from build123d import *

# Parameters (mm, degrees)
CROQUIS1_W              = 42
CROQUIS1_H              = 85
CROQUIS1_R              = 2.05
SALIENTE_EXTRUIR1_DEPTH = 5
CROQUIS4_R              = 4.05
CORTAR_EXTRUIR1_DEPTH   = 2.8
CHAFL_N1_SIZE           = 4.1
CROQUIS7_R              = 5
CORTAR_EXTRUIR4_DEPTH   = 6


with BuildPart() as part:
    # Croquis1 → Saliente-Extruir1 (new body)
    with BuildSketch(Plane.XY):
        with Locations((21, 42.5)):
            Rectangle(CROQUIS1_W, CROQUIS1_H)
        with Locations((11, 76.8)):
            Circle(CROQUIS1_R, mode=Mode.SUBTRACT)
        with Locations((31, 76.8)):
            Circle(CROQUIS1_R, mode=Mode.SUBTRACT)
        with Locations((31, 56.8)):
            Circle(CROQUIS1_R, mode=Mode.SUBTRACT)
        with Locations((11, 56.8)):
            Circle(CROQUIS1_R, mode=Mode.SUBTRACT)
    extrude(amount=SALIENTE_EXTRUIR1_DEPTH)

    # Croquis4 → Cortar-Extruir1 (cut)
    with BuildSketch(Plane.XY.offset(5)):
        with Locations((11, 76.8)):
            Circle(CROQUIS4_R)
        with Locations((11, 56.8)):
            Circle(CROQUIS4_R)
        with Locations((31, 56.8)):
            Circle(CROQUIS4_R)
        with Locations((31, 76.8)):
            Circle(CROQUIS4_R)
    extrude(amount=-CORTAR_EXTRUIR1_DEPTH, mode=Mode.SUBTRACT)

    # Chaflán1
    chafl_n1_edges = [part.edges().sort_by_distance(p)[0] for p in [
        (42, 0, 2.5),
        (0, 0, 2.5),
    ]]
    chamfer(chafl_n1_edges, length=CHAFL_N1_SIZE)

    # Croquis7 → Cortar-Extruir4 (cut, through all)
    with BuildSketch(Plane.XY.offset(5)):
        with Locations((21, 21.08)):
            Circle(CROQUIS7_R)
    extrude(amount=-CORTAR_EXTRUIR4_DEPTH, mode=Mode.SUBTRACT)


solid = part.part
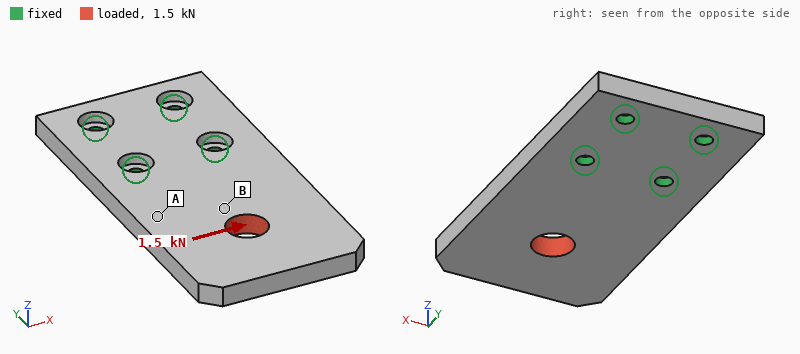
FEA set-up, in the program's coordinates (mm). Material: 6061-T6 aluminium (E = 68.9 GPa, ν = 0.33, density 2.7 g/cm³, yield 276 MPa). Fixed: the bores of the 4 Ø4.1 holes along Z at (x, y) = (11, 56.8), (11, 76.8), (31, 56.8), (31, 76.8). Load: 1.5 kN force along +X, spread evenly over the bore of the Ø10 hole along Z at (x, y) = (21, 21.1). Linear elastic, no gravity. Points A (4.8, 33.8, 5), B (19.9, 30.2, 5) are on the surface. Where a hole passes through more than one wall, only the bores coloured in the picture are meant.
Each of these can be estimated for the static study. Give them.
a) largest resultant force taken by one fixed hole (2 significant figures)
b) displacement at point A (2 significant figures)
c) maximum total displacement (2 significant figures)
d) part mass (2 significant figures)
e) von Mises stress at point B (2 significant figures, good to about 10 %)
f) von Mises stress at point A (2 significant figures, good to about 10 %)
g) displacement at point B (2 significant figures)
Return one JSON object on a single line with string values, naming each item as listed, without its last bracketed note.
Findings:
{"largest resultant force taken by one fixed hole": "1.7 kN", "displacement at point A": "24 µm", "maximum total displacement": "55 µm", "part mass": "45 g", "von Mises stress at point B": "23 MPa", "von Mises stress at point A": "11 MPa", "displacement at point B": "24 µm"}
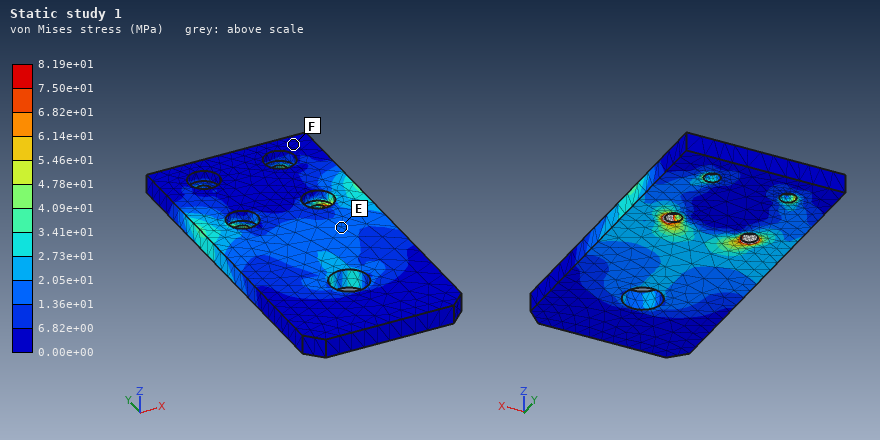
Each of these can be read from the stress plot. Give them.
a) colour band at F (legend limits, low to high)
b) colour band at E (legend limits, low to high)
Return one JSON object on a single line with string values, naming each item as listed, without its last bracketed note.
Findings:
{"colour band at F": "0.00e+00 to 6.82e+00 MPa", "colour band at E": "1.36e+01 to 2.05e+01 MPa"}
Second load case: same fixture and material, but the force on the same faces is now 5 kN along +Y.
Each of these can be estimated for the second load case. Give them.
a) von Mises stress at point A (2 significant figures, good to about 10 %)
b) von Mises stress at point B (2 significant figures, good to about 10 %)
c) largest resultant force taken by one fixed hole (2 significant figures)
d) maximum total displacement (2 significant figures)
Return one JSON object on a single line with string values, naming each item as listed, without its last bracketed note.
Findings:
{"von Mises stress at point A": "19 MPa", "von Mises stress at point B": "35 MPa", "largest resultant force taken by one fixed hole": "1.8 kN", "maximum total displacement": "80 µm"}
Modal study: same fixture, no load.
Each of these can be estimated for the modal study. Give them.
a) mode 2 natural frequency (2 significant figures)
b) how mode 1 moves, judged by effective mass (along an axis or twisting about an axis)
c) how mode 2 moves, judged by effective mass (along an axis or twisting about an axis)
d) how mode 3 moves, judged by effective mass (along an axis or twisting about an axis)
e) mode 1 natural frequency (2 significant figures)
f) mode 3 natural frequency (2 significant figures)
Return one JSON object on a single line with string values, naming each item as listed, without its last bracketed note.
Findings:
{"mode 2 natural frequency": "3400 Hz", "how mode 1 moves, judged by effective mass": "along Z", "how mode 2 moves, judged by effective mass": "twisting about Y", "how mode 3 moves, judged by effective mass": "along X", "mode 1 natural frequency": "1100 Hz", "mode 3 natural frequency": "6400 Hz"}
